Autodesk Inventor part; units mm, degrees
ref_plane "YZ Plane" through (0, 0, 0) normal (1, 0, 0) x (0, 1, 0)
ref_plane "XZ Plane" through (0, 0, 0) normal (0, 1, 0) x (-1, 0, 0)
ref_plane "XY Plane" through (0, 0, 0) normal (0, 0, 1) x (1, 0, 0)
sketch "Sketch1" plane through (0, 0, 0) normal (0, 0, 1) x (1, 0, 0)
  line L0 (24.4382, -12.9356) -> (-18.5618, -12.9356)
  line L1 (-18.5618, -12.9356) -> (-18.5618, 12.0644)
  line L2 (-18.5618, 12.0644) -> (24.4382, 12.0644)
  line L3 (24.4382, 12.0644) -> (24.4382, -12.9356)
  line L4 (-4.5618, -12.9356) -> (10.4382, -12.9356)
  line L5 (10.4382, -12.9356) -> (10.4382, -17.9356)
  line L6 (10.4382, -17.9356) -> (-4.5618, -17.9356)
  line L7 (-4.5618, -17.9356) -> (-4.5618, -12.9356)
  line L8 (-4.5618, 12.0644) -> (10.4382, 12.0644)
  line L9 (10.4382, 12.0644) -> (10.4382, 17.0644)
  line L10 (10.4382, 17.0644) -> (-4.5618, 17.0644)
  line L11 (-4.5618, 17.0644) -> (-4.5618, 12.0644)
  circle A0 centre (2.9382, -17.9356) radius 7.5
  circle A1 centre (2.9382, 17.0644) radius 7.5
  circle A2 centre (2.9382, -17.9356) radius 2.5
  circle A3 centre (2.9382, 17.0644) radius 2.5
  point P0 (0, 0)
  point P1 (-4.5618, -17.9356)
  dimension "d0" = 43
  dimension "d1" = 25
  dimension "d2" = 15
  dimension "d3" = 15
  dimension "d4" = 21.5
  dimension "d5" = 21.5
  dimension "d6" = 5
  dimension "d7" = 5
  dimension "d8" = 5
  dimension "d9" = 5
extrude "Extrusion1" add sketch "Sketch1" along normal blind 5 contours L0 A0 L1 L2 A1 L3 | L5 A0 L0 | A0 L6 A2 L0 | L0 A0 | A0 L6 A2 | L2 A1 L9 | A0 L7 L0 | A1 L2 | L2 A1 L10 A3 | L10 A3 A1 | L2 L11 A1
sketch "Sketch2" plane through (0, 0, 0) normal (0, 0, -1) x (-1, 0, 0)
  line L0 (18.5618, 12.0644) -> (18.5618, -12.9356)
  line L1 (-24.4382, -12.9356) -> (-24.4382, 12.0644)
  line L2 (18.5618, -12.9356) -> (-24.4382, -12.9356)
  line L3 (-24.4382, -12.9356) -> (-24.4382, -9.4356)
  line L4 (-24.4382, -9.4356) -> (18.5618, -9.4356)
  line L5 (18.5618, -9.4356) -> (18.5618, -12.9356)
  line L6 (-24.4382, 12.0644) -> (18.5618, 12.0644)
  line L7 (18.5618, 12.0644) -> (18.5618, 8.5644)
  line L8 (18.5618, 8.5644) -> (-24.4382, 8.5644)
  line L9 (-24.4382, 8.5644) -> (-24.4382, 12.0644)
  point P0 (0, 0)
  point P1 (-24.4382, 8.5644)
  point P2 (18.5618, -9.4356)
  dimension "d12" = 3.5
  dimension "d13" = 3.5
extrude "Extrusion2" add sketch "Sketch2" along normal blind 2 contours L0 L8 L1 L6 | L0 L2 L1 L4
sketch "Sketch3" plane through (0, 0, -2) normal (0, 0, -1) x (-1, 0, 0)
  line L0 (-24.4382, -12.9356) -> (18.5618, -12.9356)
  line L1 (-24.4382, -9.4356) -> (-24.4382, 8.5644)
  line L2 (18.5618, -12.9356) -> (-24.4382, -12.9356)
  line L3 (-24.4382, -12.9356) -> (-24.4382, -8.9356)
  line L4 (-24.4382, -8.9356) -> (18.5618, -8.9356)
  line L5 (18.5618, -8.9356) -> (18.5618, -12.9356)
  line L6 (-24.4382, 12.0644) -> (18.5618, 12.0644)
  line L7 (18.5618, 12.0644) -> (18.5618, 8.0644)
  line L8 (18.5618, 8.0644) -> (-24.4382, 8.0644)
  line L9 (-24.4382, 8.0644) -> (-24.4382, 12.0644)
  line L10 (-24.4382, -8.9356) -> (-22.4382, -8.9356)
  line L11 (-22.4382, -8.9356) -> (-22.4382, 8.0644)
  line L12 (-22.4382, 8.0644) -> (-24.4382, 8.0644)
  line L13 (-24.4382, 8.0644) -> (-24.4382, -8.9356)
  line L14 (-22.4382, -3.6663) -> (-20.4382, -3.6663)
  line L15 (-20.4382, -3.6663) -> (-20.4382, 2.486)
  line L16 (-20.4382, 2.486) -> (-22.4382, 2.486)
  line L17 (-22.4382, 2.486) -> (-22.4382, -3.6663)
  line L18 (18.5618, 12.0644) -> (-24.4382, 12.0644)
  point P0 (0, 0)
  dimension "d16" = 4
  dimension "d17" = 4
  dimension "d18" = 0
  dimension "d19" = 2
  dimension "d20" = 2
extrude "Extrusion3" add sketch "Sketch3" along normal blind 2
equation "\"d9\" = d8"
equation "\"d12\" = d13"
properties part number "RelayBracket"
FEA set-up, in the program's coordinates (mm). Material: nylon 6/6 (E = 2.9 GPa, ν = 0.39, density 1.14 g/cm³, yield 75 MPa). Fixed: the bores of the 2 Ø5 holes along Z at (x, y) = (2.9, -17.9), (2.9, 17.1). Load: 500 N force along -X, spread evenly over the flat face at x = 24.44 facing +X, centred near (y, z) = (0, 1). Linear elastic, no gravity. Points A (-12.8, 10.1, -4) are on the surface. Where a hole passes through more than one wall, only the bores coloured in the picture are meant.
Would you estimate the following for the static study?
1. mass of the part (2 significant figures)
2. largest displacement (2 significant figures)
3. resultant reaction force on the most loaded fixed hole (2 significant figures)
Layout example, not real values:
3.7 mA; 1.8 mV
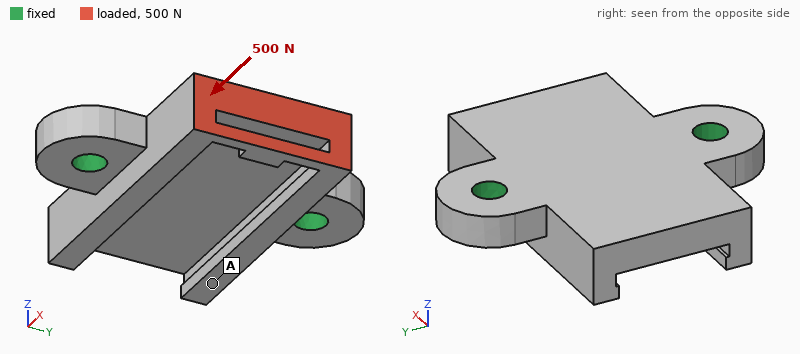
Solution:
9.3 g; 0.44 mm; 250 N
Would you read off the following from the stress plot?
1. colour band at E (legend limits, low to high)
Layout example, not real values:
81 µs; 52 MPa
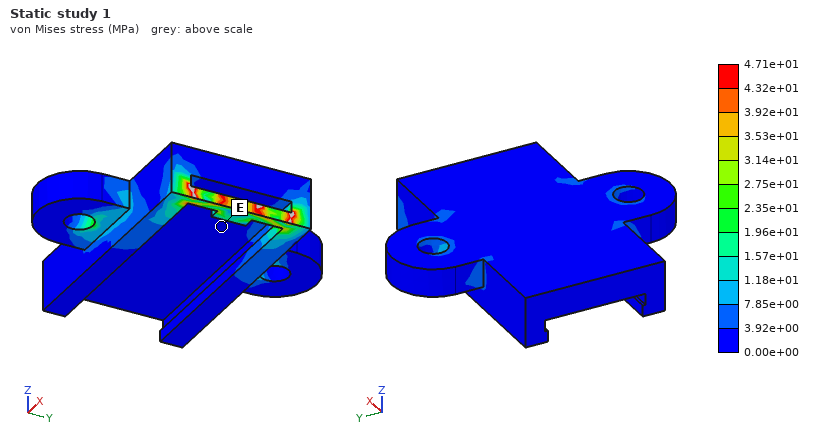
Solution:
0.00e+00 to 3.92e+00 MPa
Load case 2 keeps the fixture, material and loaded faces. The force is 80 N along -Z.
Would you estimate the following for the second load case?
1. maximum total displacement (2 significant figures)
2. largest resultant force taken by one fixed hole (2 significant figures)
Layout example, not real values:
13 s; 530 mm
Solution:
0.37 mm; 42 N
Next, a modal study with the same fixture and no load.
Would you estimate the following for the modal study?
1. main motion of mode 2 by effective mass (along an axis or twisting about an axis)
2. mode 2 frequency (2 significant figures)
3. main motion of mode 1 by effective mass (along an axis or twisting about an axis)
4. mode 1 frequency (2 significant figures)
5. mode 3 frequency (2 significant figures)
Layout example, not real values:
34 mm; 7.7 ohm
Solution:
along Z; 3300 Hz; twisting about Y; 2000 Hz; 4900 Hz
